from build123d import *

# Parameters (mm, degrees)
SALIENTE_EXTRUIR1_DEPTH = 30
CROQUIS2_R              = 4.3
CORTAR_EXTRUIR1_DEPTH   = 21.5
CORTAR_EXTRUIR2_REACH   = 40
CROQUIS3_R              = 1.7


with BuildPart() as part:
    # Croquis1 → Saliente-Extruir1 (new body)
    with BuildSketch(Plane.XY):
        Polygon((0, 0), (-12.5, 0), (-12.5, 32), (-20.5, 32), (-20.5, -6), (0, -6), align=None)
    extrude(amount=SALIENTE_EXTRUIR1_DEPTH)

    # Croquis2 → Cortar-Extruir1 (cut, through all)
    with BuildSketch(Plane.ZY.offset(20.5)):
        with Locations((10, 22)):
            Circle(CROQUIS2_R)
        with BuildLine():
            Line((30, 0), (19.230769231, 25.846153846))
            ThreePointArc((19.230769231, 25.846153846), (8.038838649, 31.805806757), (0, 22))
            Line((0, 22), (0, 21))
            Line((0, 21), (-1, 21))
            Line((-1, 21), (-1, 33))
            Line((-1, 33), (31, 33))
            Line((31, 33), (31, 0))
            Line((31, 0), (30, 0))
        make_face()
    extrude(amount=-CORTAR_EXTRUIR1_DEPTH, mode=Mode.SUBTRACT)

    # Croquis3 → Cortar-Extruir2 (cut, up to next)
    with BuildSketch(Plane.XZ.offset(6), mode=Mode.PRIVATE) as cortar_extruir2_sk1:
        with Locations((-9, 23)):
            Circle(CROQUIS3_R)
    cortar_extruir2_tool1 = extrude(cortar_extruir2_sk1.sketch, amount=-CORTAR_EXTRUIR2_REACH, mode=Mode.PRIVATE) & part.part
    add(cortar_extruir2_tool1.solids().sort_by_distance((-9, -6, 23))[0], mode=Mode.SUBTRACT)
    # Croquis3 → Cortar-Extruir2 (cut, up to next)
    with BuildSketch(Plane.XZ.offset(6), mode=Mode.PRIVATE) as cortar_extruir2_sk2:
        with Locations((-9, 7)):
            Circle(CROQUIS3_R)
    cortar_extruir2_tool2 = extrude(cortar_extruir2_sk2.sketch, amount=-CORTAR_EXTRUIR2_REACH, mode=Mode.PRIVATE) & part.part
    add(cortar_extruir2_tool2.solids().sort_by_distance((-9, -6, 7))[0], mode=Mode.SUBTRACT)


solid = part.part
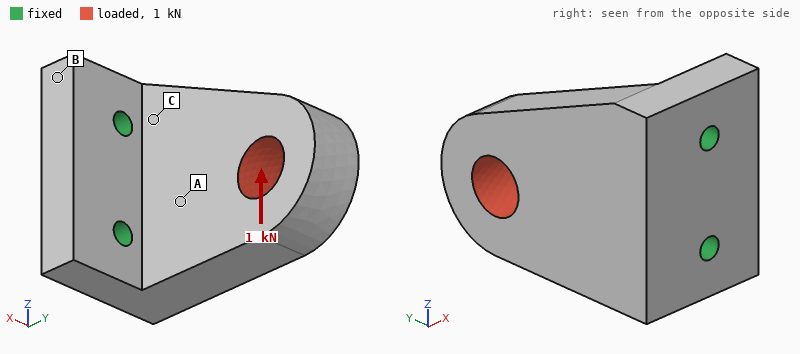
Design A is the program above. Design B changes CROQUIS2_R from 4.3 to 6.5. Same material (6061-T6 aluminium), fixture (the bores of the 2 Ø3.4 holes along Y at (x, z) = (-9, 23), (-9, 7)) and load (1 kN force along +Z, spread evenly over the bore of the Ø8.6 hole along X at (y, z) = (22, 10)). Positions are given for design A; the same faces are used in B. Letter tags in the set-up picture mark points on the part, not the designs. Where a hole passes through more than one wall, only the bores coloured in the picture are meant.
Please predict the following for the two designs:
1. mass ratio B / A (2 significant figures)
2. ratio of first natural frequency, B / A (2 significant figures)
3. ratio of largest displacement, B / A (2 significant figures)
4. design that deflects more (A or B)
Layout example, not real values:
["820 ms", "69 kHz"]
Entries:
["0.93", "1.1", "1.2", "B"]
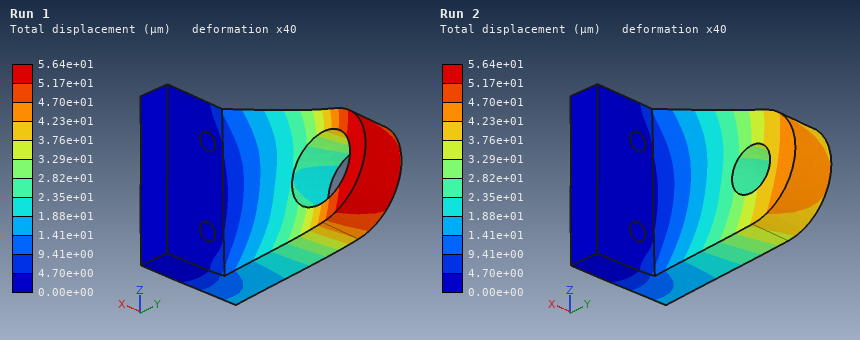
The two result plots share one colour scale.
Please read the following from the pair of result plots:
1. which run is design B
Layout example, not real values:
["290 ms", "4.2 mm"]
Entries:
["Run 1"]
